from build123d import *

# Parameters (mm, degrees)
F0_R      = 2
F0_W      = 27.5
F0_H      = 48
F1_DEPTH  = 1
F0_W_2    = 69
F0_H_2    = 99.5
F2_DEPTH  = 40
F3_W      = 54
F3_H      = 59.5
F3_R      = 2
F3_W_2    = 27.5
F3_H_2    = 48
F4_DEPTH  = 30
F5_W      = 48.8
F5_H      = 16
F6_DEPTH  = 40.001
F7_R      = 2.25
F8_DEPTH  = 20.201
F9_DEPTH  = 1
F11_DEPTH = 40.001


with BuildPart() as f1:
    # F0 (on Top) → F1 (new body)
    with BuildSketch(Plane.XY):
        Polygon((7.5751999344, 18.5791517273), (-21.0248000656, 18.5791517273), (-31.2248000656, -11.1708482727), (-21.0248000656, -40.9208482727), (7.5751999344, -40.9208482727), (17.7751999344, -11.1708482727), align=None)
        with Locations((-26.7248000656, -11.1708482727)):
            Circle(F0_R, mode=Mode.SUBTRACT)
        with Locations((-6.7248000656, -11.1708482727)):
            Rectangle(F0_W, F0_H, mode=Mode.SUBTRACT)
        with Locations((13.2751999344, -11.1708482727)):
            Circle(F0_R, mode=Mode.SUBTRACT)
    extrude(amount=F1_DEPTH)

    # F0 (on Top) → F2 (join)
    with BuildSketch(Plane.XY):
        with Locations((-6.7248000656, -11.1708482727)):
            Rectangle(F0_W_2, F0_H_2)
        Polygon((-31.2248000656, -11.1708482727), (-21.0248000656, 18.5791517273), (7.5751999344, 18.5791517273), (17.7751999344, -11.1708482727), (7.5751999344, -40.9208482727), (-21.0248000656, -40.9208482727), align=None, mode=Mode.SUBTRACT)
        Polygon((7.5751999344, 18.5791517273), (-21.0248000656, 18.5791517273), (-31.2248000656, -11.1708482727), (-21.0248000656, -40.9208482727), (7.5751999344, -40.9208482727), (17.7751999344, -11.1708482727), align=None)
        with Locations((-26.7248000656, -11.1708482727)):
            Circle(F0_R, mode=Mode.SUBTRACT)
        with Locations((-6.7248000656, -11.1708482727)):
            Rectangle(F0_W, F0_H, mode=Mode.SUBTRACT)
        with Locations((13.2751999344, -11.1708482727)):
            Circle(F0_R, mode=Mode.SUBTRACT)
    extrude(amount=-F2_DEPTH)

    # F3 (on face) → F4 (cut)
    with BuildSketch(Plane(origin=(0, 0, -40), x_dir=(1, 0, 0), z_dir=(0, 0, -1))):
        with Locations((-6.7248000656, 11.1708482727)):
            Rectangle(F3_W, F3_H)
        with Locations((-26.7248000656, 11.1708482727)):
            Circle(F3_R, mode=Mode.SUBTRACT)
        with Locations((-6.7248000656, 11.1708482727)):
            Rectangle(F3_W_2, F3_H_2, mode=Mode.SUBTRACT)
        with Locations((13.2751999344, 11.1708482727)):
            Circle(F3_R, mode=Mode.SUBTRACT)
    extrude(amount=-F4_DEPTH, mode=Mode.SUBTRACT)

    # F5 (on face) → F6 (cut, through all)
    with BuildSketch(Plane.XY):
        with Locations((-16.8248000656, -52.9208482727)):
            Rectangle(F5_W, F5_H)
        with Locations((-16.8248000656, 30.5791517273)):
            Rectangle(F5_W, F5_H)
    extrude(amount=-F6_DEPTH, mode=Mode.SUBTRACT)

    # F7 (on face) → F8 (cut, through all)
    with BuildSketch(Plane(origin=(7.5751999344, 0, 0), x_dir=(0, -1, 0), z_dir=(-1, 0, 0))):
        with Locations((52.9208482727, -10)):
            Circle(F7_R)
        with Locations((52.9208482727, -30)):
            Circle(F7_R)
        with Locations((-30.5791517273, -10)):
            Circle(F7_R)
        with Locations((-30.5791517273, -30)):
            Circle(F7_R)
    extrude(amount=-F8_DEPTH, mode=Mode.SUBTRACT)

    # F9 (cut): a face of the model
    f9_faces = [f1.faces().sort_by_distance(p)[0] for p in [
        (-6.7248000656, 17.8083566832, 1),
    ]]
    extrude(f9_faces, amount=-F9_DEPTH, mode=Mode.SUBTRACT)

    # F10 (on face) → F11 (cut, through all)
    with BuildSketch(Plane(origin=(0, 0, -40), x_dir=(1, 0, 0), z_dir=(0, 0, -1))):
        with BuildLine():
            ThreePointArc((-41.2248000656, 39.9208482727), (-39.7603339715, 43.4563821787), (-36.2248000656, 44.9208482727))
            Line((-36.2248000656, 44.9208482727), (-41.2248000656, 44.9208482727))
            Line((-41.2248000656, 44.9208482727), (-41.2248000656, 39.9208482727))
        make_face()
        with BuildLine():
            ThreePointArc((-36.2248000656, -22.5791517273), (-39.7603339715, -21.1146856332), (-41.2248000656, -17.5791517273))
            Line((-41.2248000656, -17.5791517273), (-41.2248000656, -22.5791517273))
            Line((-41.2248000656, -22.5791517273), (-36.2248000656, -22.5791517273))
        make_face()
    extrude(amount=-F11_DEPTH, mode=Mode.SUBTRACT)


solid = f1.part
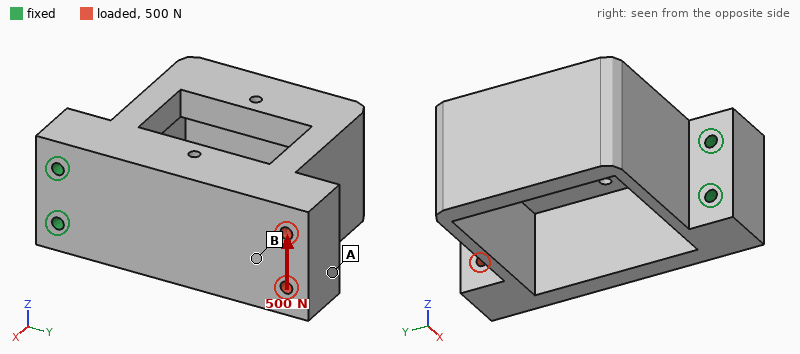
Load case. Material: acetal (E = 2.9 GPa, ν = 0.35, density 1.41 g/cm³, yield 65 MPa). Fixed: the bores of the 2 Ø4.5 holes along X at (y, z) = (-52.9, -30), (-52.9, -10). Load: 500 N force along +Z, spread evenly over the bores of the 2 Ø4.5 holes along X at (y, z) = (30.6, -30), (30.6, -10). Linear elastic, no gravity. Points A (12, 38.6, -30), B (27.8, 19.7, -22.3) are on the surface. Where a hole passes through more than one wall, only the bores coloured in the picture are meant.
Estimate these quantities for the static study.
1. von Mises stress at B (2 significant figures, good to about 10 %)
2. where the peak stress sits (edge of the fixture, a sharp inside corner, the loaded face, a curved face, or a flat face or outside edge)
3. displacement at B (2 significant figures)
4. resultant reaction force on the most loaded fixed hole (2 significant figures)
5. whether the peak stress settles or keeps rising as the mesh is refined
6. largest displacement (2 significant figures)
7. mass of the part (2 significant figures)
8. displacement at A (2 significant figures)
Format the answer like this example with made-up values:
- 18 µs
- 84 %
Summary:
- 3.3 MPa
- edge of the fixture
- 0.74 mm
- 1.8 kN
- keeps rising
- 1.3 mm
- 140 g
- 1.1 mm
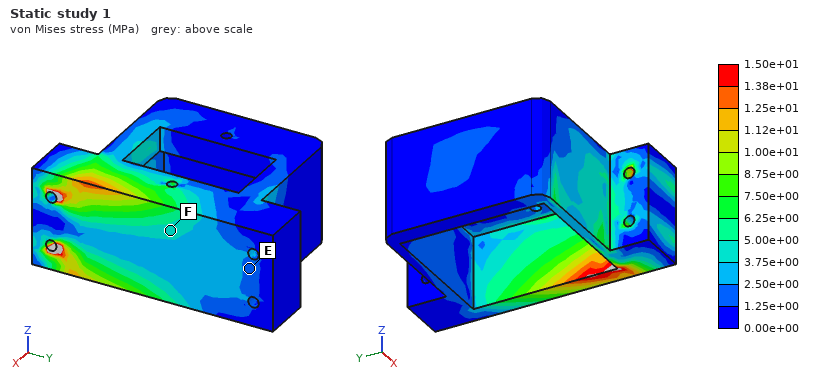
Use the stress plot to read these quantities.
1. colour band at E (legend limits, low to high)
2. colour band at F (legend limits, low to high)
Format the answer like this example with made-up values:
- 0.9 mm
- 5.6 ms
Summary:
- 1.25e+00 to 2.50e+00 MPa
- 3.75e+00 to 5.00e+00 MPa
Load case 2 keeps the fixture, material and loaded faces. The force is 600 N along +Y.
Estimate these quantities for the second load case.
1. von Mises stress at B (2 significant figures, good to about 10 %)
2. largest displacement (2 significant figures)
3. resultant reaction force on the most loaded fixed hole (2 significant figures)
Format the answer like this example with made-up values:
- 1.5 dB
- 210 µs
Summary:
- 1.1 MPa
- 0.31 mm
- 300 N
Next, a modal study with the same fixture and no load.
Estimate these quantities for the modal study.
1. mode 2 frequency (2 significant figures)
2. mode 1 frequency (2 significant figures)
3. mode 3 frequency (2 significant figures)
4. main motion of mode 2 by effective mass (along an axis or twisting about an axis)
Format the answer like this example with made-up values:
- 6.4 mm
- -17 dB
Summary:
- 350 Hz
- 260 Hz
- 740 Hz
- along Z
